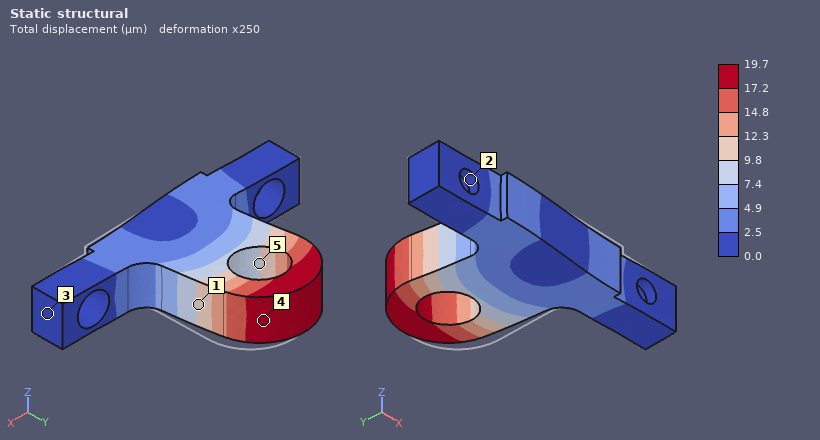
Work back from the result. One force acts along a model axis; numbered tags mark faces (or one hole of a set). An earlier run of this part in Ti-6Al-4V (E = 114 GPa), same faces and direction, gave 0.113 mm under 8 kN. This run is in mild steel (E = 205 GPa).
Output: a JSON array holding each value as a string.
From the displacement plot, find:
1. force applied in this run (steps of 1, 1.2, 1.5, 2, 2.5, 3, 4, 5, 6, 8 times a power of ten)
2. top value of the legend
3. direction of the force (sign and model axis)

["2.5 kN", "19.7 µm", "-X"]
